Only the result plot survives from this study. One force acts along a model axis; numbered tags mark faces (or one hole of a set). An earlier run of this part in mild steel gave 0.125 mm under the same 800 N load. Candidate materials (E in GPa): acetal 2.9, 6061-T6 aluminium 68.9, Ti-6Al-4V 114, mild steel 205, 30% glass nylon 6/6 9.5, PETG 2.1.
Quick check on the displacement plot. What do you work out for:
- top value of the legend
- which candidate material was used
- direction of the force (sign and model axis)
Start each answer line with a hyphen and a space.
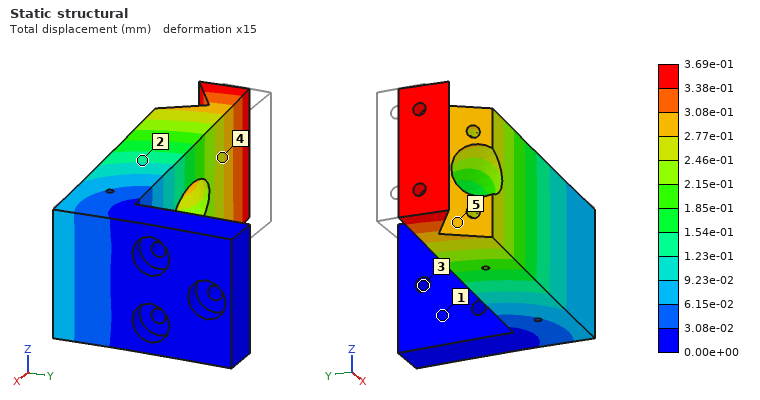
- 3.69e-01 mm
- 6061-T6 aluminium
- -Y
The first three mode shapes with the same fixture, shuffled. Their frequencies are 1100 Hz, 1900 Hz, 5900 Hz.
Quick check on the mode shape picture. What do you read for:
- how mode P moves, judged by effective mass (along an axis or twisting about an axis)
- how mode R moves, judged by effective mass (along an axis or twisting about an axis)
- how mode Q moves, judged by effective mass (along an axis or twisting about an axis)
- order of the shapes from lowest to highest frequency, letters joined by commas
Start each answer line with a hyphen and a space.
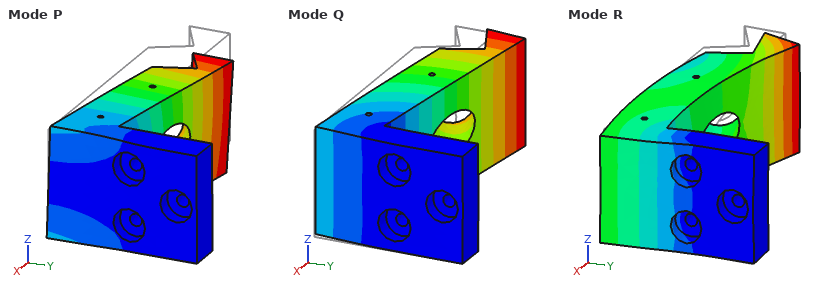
- along Z
- along X
- along Y
- Q, P, R
